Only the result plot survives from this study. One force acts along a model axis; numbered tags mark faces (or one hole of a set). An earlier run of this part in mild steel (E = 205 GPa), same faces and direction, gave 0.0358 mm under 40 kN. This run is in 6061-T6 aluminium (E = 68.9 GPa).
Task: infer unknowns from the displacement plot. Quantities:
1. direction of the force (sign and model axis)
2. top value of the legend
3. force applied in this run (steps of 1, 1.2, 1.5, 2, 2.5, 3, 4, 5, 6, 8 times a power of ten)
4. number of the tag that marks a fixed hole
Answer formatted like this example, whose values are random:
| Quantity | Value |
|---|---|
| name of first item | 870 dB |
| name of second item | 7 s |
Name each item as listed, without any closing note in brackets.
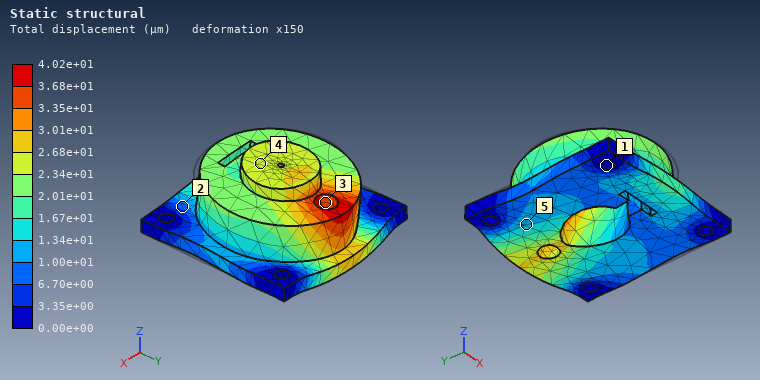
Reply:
| Quantity | Value |
|---|---|
| direction of the force | +Y |
| top value of the legend | 4.02e+01 µm |
| force applied in this run | 15 kN |
| number of the tag that marks a fixed hole | 1 |
